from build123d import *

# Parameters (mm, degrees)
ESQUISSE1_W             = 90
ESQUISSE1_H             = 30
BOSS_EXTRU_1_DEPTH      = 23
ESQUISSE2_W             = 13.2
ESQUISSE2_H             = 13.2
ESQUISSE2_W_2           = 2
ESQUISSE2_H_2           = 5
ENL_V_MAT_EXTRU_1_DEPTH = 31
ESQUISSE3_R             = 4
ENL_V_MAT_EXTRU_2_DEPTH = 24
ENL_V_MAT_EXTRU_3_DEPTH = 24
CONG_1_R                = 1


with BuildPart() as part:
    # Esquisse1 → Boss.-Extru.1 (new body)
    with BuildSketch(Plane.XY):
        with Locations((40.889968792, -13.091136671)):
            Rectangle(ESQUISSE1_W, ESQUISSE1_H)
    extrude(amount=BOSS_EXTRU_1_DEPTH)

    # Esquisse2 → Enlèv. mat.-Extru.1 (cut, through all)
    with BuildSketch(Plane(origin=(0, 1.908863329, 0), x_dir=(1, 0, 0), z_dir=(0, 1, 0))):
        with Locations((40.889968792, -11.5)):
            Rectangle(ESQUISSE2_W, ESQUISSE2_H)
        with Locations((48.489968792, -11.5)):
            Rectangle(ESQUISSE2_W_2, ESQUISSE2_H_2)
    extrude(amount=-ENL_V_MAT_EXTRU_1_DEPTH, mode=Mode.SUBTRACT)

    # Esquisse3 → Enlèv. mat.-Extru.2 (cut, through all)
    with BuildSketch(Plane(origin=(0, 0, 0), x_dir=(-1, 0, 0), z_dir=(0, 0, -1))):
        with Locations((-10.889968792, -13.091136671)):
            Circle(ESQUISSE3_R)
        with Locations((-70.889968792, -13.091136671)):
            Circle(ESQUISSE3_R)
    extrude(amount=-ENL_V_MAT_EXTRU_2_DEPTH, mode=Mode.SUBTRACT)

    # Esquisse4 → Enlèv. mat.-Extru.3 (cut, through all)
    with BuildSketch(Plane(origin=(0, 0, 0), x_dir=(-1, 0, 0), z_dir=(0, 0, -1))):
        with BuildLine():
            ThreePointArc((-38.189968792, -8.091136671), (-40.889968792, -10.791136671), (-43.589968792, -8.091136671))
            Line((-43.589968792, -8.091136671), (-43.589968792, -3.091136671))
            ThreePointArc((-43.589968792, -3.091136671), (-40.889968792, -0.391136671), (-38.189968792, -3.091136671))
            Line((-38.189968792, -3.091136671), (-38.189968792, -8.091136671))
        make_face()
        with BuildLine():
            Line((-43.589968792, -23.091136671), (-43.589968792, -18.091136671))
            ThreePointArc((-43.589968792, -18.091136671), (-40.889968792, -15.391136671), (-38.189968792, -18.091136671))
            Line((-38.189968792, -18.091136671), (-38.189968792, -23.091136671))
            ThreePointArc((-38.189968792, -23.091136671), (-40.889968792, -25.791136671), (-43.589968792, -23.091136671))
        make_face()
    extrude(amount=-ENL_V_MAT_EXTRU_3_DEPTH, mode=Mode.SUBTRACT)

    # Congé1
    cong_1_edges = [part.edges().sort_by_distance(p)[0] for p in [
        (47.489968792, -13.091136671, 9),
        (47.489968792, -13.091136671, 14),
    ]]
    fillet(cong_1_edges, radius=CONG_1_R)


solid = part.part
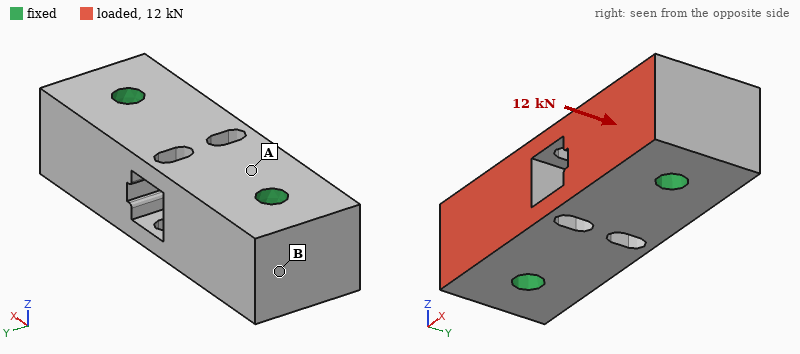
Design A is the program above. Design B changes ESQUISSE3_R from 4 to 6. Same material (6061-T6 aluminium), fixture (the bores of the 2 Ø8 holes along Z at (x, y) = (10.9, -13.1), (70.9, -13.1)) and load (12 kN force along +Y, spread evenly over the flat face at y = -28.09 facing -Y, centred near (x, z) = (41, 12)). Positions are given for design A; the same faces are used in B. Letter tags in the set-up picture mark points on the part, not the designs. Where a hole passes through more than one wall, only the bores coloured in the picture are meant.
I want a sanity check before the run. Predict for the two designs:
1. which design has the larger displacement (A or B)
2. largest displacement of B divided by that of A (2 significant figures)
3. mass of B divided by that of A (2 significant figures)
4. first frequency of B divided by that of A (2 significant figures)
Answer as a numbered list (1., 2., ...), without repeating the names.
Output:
1. A
2. 0.78
3. 0.95
4. 1.3
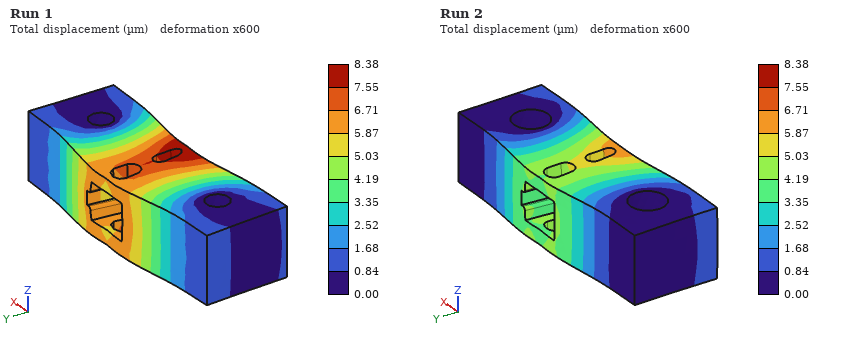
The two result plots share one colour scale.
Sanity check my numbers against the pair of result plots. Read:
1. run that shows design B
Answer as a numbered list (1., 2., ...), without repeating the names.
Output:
1. Run 2
